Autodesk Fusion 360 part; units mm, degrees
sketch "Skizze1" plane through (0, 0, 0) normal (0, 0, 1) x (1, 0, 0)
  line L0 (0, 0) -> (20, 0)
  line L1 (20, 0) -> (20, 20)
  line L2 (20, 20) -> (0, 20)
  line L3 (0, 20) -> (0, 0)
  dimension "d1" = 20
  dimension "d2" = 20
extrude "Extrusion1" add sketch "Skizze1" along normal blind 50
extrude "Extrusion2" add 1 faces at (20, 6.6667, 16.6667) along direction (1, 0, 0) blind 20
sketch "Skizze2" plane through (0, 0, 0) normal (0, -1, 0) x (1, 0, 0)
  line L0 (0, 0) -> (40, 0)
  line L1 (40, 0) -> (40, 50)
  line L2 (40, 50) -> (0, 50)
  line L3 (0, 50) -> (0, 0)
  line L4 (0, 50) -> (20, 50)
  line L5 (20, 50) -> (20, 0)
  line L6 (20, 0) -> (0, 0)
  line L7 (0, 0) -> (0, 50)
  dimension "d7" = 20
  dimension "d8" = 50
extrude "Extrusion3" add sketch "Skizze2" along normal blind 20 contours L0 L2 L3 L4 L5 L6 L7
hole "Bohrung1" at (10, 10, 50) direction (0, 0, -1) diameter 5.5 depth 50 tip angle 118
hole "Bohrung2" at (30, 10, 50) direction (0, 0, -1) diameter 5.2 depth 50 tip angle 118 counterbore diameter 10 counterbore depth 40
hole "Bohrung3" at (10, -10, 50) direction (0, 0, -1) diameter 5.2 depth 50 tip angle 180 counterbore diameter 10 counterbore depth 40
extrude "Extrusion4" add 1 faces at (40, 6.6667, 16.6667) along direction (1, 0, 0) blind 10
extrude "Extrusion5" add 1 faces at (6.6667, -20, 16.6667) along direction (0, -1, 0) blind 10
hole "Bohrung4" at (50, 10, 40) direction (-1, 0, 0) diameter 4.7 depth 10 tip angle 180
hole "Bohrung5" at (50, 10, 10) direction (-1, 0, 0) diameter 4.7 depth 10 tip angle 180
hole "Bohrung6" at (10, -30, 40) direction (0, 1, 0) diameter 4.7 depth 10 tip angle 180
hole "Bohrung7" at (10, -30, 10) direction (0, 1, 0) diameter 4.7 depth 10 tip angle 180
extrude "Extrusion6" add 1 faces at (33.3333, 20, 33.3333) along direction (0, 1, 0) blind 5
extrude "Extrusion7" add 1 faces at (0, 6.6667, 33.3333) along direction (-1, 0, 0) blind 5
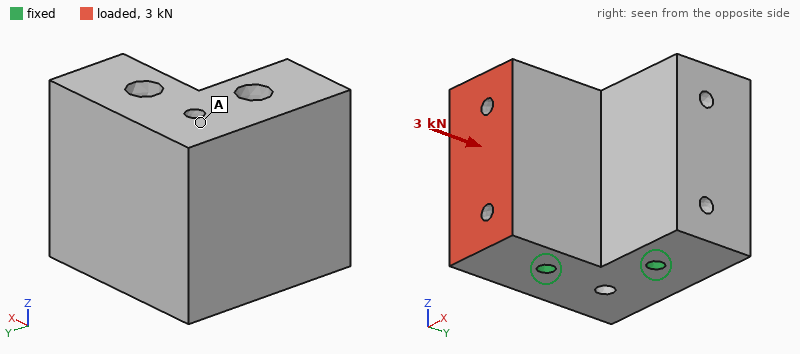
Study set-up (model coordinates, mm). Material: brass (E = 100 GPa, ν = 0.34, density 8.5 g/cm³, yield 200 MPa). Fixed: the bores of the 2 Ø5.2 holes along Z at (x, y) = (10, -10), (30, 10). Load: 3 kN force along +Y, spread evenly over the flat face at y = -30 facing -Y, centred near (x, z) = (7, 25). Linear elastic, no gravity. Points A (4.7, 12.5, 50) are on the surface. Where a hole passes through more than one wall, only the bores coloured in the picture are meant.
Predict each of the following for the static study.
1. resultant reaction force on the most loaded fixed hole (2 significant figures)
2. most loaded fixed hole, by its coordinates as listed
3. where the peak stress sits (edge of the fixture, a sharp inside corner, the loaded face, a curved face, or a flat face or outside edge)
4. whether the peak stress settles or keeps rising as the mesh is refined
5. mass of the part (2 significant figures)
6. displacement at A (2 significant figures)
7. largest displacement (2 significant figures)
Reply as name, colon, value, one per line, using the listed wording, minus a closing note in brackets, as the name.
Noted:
resultant reaction force on the most loaded fixed hole: 2.9 kN
most loaded fixed hole, by its coordinates as listed: (10, -10)
where the peak stress sits: edge of the fixture
whether the peak stress settles or keeps rising as the mesh is refined: keeps rising
mass of the part: 830 g
displacement at A: 25 µm
largest displacement: 29 µm
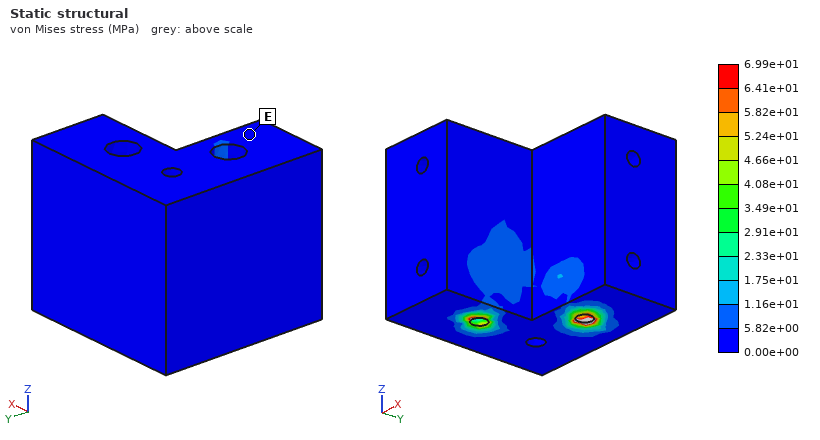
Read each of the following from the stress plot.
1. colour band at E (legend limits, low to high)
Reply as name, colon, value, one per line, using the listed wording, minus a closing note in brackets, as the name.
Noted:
colour band at E: 0.00e+00 to 5.82e+00 MPa
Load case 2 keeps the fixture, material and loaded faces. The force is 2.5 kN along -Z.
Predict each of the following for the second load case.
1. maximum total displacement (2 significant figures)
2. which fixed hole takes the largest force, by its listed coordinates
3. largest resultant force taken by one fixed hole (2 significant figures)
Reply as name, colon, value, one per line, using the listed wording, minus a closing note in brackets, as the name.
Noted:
maximum total displacement: 22 µm
which fixed hole takes the largest force, by its listed coordinates: (10, -10)
largest resultant force taken by one fixed hole: 3.5 kN
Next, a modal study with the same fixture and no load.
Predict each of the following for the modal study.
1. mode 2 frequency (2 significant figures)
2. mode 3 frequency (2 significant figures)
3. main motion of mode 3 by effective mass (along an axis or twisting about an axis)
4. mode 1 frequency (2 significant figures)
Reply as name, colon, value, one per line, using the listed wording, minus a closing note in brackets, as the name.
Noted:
mode 2 frequency: 3700 Hz
mode 3 frequency: 5000 Hz
main motion of mode 3 by effective mass: twisting about Z
mode 1 frequency: 1900 Hz
